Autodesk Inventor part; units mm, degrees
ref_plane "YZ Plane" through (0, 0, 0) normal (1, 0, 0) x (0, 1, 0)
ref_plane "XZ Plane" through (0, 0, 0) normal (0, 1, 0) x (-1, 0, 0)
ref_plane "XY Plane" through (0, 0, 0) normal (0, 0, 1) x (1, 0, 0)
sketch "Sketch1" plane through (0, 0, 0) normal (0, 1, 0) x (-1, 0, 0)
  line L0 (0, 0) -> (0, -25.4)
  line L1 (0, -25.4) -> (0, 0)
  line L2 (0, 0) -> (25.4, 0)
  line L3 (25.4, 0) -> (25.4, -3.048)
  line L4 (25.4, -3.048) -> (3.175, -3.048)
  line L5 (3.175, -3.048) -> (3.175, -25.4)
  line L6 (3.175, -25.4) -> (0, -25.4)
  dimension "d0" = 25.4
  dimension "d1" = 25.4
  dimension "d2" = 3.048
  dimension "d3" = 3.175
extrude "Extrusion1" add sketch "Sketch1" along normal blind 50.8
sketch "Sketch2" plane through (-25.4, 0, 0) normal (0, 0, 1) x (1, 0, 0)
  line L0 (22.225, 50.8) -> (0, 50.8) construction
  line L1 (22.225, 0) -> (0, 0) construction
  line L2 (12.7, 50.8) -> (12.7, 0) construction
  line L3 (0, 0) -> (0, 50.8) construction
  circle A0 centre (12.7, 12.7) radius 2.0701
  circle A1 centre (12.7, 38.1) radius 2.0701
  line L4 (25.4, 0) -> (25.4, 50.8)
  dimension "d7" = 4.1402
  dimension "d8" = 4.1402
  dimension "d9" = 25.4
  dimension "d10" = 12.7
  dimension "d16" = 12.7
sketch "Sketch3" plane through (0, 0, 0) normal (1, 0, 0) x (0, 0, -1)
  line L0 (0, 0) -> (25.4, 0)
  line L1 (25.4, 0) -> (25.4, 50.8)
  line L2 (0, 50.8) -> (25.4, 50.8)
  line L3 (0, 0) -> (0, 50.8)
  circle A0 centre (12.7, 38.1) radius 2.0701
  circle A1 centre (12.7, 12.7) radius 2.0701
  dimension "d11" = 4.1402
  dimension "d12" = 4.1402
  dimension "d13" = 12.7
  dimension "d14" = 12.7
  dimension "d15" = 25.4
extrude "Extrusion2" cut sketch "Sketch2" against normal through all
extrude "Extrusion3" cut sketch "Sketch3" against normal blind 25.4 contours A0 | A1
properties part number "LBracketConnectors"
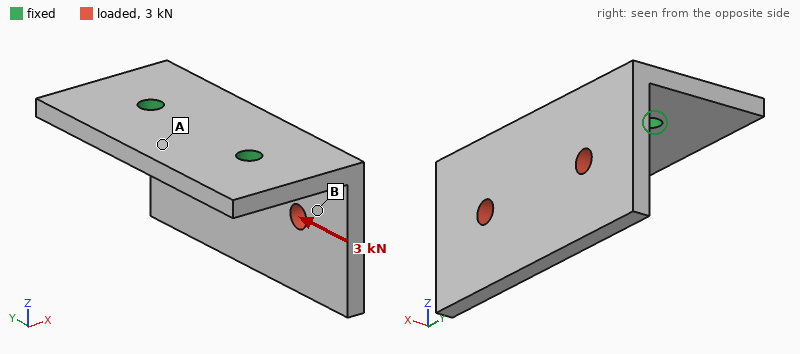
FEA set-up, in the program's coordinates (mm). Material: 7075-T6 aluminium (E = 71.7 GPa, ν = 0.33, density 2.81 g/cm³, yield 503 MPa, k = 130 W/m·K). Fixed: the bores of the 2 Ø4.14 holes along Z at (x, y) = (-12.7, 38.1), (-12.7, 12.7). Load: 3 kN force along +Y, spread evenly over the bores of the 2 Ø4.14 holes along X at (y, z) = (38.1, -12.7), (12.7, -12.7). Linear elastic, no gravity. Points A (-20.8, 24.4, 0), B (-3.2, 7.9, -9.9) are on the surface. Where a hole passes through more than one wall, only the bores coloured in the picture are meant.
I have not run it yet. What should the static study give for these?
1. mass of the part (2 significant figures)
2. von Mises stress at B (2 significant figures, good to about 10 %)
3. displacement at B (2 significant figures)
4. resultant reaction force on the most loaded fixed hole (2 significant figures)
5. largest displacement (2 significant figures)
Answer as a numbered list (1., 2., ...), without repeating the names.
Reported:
1. 21 g
2. 78 MPa
3. 0.13 mm
4. 2.2 kN
5. 0.26 mm
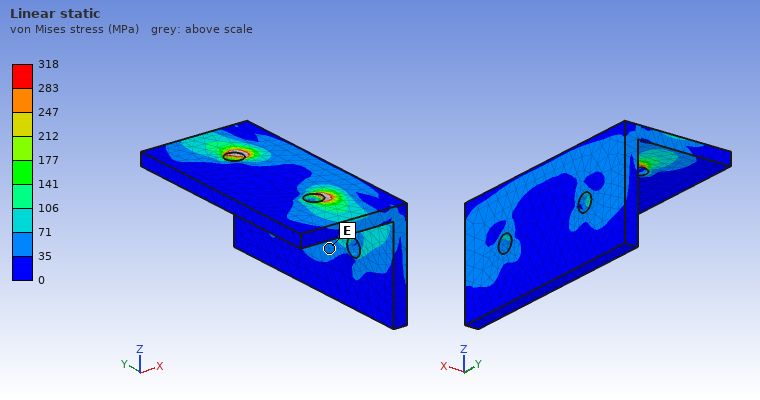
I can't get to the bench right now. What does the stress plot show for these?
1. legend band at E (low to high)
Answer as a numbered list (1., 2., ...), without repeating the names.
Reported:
1. 35 to 71 MPa
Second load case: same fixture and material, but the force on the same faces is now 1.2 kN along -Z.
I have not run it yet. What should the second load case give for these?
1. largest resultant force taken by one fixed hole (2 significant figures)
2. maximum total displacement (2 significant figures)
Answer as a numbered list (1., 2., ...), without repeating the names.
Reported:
1. 600 N
2. 0.23 mm
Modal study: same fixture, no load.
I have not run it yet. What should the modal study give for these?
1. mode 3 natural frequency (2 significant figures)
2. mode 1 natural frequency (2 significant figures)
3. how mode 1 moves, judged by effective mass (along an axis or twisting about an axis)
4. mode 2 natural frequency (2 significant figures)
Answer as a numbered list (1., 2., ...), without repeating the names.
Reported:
1. 7100 Hz
2. 2600 Hz
3. along X
4. 4400 Hz
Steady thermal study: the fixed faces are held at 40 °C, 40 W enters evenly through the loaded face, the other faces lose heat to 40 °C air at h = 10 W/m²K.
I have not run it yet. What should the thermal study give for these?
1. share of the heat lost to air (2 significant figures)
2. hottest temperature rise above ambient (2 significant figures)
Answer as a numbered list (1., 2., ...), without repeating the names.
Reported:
1. 3.4 %
2. 54 K
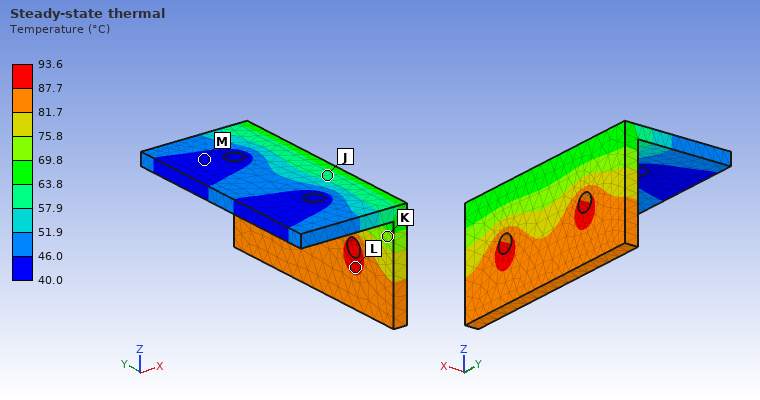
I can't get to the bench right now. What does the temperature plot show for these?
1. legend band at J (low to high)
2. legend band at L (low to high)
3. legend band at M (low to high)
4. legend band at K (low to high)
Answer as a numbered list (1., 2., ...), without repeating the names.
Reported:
1. 57.9 to 63.8 °C
2. 87.7 to 93.6 °C
3. 40.0 to 46.0 °C
4. 69.8 to 75.8 °C
